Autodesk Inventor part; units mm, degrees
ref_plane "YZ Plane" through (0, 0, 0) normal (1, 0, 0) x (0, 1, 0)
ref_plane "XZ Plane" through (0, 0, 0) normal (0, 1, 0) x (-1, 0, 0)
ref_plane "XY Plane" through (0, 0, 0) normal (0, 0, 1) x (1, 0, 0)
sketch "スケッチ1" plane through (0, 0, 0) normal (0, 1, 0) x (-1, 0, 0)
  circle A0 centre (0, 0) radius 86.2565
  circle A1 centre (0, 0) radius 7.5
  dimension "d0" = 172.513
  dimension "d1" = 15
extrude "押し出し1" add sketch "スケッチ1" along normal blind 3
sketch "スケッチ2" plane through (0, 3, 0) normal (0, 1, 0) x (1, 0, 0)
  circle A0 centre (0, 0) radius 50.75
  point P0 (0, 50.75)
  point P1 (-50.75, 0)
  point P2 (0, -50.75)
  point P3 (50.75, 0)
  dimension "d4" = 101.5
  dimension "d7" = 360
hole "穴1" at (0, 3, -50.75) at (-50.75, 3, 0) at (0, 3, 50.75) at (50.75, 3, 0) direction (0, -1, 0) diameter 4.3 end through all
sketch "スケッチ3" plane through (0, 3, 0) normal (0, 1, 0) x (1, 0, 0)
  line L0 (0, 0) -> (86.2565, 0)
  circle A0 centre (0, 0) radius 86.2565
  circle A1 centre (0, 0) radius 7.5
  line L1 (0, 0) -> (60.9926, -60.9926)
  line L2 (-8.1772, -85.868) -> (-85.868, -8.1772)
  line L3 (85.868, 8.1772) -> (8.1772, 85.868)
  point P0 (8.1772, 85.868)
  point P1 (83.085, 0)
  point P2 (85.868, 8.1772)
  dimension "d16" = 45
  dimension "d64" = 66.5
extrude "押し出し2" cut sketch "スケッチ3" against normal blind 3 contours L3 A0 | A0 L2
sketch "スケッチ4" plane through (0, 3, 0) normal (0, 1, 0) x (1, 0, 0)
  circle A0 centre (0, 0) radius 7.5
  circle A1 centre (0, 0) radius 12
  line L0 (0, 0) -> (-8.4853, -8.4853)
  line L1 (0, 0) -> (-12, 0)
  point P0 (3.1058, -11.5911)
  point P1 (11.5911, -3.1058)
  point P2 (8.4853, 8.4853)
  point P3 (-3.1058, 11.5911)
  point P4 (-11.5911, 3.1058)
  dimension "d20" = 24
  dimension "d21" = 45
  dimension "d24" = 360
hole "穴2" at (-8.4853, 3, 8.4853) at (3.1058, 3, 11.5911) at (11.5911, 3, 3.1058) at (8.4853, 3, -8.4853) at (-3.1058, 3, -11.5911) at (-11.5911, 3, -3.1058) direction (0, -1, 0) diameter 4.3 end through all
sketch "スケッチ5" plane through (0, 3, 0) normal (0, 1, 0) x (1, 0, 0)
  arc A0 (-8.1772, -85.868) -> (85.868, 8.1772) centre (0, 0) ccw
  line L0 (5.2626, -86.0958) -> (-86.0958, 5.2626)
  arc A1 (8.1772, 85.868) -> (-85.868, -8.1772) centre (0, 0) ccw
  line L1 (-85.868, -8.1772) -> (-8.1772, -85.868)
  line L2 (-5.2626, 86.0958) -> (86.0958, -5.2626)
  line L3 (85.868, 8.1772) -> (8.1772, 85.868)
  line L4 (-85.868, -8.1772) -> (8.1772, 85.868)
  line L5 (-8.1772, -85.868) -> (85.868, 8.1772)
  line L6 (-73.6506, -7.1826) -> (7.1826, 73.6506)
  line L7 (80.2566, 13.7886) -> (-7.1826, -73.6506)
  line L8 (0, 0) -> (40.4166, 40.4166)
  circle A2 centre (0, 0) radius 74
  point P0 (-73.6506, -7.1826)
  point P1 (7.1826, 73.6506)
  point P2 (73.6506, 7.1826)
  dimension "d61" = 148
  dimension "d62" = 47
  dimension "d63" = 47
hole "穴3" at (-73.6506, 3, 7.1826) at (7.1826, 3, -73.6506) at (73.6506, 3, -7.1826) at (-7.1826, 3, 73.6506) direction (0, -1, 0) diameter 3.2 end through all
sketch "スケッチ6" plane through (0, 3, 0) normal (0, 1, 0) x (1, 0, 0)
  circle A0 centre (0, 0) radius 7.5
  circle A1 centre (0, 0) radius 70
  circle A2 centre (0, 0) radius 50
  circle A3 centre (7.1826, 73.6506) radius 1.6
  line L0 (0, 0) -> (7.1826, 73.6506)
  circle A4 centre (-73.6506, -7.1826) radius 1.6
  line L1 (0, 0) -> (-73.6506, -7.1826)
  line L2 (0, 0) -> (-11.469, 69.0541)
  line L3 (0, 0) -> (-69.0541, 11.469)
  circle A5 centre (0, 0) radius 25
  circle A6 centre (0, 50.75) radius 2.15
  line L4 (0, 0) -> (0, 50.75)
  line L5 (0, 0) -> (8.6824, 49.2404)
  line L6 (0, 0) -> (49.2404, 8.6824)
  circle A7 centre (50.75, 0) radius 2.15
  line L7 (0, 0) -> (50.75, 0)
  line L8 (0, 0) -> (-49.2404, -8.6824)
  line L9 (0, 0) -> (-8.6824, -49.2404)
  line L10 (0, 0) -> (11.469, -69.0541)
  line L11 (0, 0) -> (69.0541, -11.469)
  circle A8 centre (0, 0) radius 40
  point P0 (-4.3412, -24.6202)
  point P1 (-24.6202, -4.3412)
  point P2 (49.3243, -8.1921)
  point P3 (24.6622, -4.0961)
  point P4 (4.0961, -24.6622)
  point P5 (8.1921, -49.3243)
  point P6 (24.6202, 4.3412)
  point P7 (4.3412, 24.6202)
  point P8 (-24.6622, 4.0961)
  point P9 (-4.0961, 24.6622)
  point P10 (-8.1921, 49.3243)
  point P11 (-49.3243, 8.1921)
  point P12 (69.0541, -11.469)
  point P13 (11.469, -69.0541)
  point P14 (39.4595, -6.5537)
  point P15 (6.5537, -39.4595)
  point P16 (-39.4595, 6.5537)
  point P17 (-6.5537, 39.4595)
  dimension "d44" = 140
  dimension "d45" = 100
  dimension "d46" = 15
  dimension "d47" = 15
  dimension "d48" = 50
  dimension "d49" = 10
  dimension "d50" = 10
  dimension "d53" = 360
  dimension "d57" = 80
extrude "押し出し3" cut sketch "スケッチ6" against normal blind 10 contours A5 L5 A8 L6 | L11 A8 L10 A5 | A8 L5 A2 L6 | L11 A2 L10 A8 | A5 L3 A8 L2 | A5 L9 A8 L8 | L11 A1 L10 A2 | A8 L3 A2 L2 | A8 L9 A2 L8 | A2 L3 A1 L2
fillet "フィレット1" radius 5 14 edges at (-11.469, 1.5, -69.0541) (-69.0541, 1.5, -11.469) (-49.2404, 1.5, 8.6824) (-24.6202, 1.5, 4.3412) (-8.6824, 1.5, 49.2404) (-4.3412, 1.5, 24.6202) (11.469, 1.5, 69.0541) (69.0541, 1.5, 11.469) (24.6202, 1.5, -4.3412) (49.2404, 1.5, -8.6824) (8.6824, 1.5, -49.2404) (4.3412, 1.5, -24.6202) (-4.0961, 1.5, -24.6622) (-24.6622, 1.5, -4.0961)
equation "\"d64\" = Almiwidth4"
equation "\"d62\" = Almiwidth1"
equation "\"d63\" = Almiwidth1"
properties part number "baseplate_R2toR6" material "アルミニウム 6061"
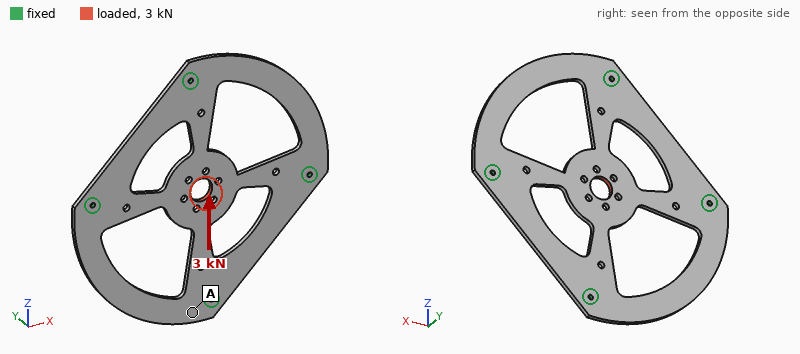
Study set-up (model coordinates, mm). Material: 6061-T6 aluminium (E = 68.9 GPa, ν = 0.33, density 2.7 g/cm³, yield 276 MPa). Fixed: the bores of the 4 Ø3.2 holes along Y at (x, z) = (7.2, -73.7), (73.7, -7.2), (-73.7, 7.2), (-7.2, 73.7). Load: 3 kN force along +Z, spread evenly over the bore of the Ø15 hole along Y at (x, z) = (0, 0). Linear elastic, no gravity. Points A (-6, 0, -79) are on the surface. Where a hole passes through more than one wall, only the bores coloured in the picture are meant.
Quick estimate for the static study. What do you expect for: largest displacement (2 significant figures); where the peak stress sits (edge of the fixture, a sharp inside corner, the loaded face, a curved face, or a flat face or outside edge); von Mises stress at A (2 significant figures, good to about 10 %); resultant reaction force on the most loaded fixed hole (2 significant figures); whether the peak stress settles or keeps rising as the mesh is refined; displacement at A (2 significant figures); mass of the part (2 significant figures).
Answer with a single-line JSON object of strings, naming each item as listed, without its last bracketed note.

{"largest displacement": "36 µm", "where the peak stress sits": "edge of the fixture", "von Mises stress at A": "7.2 MPa", "resultant reaction force on the most loaded fixed hole": "1.3 kN", "whether the peak stress settles or keeps rising as the mesh is refined": "keeps rising", "displacement at A": "5.8 µm", "mass of the part": "100 g"}
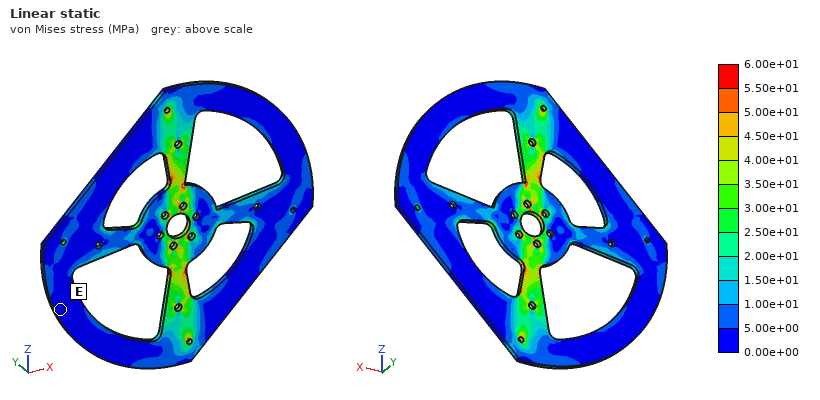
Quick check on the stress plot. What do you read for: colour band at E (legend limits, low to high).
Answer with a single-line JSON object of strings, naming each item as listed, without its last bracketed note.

{"colour band at E": "0.00e+00 to 5.00e+00 MPa"}
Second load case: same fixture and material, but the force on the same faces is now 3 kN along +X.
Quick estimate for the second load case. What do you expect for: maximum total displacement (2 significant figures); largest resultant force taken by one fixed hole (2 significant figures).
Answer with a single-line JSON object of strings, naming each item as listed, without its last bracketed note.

{"maximum total displacement": "36 µm", "largest resultant force taken by one fixed hole": "1.3 kN"}
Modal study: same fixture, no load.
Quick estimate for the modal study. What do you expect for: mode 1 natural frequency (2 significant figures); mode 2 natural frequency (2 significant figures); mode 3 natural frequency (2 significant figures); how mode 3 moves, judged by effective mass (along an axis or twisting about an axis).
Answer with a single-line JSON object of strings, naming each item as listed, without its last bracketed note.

{"mode 1 natural frequency": "850 Hz", "mode 2 natural frequency": "860 Hz", "mode 3 natural frequency": "920 Hz", "how mode 3 moves, judged by effective mass": "along Y"}
